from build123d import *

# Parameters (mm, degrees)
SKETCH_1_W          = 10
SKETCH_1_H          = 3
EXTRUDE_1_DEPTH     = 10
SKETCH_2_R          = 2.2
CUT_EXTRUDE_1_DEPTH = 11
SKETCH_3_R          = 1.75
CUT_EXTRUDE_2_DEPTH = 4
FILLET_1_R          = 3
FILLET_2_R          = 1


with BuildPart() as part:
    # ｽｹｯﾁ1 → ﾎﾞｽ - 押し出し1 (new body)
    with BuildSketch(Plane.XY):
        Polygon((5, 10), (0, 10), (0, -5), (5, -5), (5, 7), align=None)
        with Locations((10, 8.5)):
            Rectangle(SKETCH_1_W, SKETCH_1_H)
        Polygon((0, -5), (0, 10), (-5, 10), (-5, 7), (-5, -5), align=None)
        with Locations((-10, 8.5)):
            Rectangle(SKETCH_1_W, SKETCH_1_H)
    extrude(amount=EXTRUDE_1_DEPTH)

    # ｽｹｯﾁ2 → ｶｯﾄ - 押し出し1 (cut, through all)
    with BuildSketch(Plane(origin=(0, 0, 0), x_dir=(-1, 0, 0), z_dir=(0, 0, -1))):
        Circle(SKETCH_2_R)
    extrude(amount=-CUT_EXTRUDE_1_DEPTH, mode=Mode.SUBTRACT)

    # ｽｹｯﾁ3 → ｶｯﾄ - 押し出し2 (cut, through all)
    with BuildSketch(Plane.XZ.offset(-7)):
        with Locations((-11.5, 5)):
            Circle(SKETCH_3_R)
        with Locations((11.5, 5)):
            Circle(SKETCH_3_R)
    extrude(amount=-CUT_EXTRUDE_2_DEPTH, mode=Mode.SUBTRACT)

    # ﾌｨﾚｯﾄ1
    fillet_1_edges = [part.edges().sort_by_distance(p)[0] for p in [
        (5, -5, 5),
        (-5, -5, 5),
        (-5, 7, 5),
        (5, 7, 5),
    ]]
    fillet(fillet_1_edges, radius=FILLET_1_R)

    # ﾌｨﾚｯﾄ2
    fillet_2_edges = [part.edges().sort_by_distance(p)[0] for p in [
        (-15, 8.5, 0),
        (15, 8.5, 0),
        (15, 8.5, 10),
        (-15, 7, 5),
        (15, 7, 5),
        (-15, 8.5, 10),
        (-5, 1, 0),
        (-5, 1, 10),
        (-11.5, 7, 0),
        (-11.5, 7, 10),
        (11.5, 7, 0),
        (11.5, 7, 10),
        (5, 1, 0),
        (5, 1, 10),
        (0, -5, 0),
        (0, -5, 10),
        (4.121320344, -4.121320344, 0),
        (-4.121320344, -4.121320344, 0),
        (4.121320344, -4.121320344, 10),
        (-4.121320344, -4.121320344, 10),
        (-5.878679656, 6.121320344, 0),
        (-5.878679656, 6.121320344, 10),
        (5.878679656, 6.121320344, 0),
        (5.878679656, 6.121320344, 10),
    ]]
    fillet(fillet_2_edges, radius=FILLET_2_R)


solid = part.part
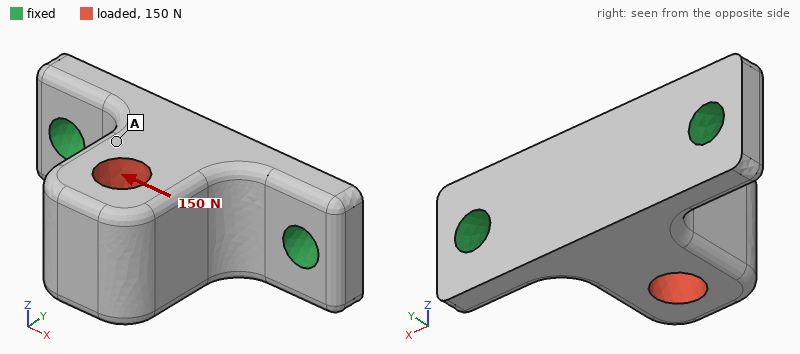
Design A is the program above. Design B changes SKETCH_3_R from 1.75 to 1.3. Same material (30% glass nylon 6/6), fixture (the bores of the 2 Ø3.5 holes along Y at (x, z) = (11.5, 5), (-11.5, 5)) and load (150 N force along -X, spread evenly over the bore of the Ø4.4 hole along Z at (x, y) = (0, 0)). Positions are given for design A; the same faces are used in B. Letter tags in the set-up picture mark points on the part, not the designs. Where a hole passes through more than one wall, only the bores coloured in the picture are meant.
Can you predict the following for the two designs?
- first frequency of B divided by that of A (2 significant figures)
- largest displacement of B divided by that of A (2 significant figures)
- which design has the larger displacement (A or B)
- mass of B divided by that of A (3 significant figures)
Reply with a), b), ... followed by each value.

a) 0.91
b) 1.1
c) B
d) 1.01
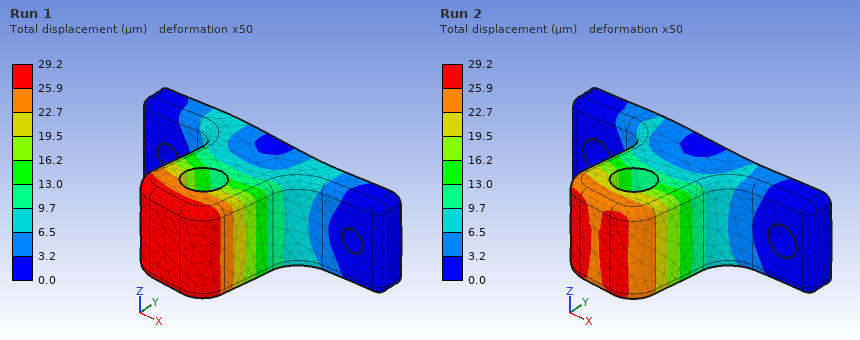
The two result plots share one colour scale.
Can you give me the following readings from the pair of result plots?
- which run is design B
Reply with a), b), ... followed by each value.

a) Run 1
